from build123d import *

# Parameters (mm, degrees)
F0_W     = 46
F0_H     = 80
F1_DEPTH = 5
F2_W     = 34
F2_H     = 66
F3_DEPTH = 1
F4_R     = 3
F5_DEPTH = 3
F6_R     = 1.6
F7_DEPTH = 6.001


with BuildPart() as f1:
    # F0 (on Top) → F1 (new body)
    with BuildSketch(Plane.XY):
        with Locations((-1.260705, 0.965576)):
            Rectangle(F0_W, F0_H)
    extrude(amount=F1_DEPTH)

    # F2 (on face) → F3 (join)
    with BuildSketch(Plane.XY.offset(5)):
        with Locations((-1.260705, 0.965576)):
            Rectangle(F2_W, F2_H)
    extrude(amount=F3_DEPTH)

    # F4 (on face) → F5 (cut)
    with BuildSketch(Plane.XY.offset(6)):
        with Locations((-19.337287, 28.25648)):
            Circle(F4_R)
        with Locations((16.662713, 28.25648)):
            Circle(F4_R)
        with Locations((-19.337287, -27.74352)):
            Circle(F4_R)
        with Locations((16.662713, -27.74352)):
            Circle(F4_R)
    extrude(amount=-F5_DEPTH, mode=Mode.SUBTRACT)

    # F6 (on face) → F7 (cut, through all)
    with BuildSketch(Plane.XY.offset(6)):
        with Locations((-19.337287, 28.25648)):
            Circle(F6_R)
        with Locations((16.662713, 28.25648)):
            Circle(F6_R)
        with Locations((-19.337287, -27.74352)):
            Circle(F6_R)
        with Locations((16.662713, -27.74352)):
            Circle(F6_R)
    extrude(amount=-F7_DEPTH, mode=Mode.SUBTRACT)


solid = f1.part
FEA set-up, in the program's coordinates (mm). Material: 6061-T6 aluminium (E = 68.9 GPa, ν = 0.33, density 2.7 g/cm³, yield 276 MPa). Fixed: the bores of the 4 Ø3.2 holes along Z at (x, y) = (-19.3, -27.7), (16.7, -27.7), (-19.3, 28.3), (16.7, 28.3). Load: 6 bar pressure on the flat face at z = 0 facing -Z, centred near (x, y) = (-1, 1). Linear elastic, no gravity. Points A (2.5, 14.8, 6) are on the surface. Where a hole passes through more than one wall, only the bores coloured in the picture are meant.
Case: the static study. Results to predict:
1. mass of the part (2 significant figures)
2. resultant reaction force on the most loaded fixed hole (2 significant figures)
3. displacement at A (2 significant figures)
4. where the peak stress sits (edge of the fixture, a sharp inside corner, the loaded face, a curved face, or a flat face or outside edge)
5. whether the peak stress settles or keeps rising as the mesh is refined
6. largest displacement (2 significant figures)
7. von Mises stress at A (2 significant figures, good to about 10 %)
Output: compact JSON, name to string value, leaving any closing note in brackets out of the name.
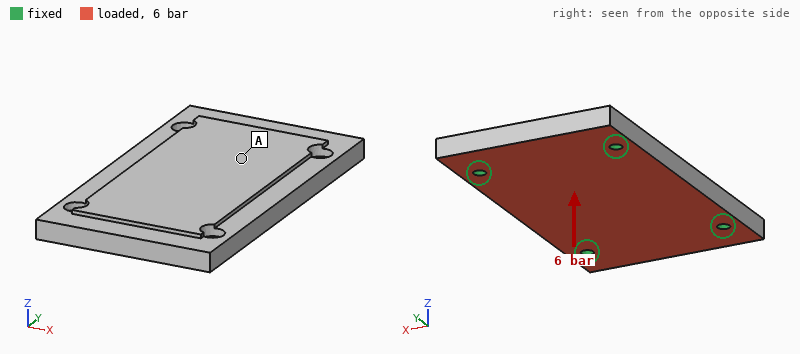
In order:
{"mass of the part": "55 g", "resultant reaction force on the most loaded fixed hole": "680 N", "displacement at A": "22 µm", "where the peak stress sits": "edge of the fixture", "whether the peak stress settles or keeps rising as the mesh is refined": "keeps rising", "largest displacement": "30 µm", "von Mises stress at A": "11 MPa"}
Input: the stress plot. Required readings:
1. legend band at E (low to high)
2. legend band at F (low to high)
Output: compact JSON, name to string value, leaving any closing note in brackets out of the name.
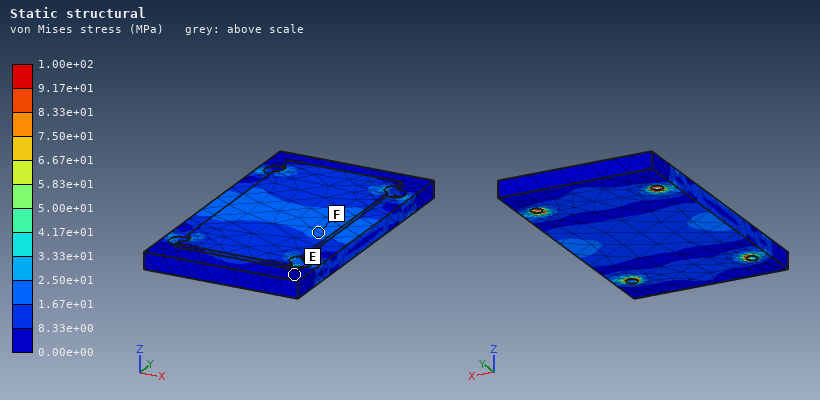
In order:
{"legend band at E": "0.00e+00 to 8.33e+00 MPa", "legend band at F": "1.67e+01 to 2.50e+01 MPa"}
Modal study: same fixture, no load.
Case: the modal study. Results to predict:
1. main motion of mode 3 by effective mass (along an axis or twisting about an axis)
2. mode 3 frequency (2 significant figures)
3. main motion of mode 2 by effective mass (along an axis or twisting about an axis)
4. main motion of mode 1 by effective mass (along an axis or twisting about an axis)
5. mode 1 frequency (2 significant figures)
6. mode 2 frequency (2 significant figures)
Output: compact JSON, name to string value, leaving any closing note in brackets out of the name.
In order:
{"main motion of mode 3 by effective mass": "along Z", "mode 3 frequency": "12 kHz", "main motion of mode 2 by effective mass": "twisting about Y", "main motion of mode 1 by effective mass": "along Z", "mode 1 frequency": "6100 Hz", "mode 2 frequency": "9800 Hz"}
